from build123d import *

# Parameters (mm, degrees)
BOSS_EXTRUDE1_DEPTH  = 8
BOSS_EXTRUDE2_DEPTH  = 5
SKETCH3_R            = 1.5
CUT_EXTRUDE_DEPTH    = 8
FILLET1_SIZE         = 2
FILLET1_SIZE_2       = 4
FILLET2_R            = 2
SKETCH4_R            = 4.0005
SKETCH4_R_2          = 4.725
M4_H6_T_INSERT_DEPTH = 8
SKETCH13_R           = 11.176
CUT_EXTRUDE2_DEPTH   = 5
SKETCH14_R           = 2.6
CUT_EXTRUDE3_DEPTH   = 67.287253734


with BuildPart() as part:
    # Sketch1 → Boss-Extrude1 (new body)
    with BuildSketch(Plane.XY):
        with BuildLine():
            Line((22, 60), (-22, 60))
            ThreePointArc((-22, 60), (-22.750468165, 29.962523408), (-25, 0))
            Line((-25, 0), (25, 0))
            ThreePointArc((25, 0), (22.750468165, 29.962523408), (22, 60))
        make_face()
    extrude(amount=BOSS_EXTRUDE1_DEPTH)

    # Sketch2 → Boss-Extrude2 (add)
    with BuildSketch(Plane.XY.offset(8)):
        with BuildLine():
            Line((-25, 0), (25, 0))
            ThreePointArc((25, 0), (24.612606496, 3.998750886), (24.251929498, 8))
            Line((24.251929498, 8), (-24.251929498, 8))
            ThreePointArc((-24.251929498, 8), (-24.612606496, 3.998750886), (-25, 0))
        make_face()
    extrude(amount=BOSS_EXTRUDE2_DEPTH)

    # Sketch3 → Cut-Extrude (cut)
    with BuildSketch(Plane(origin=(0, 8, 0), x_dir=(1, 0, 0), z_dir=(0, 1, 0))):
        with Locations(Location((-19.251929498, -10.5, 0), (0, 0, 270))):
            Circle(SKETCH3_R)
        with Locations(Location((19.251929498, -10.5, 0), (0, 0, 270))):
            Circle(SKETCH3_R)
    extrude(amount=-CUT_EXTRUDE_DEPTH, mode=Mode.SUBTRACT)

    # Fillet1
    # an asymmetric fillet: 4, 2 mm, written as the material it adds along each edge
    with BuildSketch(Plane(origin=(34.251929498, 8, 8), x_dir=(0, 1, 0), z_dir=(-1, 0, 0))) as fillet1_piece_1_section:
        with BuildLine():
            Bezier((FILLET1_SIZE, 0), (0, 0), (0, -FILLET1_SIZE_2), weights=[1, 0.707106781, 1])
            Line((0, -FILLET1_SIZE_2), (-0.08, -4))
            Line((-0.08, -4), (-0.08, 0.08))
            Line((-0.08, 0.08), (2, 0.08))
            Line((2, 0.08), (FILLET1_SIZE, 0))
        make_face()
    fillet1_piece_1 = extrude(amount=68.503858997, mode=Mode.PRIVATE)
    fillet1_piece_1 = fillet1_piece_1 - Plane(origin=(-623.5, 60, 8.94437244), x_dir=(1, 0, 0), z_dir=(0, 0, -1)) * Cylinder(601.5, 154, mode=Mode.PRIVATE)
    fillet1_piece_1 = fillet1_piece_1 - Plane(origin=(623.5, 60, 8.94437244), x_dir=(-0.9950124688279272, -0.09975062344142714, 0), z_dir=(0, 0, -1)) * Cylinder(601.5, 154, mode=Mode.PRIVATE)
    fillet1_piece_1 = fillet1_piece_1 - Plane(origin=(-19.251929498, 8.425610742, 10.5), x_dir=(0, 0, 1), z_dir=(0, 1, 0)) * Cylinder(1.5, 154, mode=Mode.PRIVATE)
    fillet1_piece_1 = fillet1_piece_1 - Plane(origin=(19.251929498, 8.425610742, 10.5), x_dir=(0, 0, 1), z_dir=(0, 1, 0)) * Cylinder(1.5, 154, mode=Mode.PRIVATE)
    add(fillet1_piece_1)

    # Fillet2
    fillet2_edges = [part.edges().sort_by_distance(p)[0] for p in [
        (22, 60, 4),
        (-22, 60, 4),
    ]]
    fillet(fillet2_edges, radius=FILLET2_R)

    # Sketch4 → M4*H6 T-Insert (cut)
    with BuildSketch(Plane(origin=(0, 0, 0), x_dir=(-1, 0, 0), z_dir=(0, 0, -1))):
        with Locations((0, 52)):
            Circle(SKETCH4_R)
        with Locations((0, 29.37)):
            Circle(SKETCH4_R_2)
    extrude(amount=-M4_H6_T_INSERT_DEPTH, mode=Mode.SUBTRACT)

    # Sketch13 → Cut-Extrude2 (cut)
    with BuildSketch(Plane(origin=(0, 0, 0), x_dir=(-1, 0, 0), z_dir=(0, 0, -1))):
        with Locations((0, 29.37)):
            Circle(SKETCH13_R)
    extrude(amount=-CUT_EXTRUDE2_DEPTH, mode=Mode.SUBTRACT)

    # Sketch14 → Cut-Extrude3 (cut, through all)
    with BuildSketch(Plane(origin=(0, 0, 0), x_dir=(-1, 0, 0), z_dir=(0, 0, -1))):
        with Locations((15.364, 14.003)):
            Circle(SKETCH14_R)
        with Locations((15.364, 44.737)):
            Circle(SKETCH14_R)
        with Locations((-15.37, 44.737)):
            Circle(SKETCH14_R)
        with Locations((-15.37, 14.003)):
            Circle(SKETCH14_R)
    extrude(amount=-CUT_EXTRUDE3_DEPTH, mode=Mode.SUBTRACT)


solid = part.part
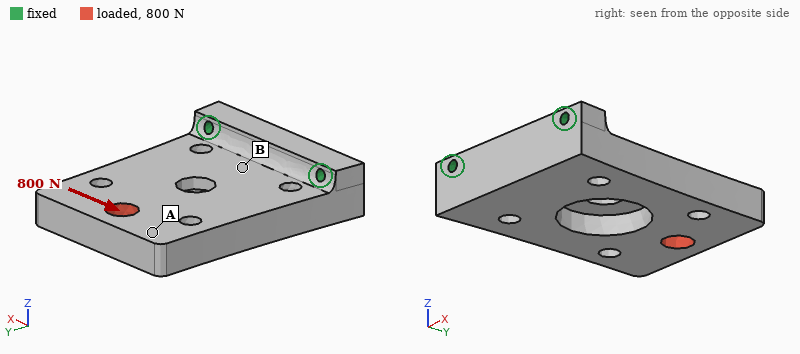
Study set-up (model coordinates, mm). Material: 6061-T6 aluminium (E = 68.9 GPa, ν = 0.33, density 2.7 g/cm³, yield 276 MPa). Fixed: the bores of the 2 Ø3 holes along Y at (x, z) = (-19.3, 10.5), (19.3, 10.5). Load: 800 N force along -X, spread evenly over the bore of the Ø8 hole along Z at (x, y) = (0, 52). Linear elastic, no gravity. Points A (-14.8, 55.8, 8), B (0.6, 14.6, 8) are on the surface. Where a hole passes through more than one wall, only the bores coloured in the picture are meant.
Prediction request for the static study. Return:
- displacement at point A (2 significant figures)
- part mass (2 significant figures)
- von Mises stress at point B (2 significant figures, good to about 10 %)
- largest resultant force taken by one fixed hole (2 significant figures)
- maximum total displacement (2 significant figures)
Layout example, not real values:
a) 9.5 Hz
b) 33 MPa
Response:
a) 25 µm
b) 56 g
c) 11 MPa
d) 1.0 kN
e) 27 µm
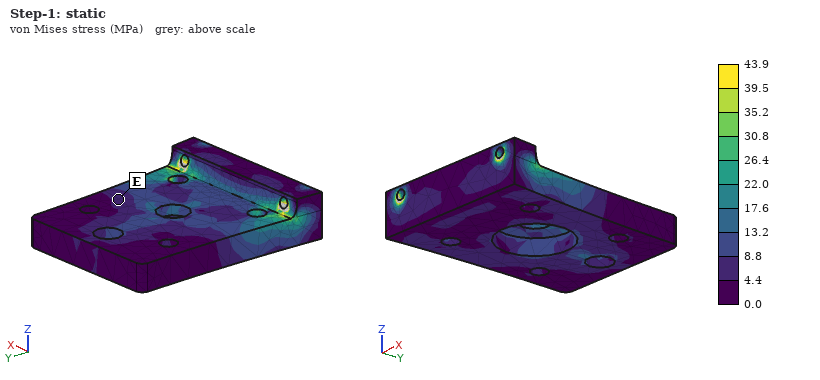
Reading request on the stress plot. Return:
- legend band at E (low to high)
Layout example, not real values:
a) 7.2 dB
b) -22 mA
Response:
a) 4.4 to 8.8 MPa
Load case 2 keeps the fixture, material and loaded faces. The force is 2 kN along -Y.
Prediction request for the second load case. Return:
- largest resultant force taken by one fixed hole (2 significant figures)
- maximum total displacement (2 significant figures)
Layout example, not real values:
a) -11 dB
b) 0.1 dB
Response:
a) 1.0 kN
b) 60 µm
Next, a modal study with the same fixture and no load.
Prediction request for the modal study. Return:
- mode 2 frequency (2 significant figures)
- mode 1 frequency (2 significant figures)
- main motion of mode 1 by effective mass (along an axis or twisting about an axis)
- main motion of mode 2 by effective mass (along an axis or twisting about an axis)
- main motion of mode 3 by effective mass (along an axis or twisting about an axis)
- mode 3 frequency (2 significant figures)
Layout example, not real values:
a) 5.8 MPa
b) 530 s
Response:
a) 4900 Hz
b) 1700 Hz
c) along Z
d) twisting about Y
e) along X
f) 6500 Hz
